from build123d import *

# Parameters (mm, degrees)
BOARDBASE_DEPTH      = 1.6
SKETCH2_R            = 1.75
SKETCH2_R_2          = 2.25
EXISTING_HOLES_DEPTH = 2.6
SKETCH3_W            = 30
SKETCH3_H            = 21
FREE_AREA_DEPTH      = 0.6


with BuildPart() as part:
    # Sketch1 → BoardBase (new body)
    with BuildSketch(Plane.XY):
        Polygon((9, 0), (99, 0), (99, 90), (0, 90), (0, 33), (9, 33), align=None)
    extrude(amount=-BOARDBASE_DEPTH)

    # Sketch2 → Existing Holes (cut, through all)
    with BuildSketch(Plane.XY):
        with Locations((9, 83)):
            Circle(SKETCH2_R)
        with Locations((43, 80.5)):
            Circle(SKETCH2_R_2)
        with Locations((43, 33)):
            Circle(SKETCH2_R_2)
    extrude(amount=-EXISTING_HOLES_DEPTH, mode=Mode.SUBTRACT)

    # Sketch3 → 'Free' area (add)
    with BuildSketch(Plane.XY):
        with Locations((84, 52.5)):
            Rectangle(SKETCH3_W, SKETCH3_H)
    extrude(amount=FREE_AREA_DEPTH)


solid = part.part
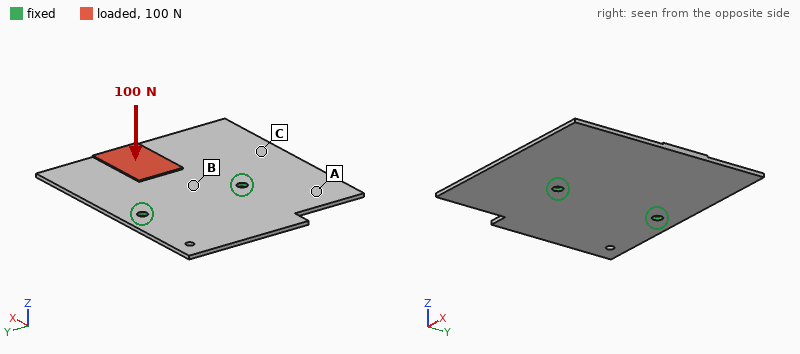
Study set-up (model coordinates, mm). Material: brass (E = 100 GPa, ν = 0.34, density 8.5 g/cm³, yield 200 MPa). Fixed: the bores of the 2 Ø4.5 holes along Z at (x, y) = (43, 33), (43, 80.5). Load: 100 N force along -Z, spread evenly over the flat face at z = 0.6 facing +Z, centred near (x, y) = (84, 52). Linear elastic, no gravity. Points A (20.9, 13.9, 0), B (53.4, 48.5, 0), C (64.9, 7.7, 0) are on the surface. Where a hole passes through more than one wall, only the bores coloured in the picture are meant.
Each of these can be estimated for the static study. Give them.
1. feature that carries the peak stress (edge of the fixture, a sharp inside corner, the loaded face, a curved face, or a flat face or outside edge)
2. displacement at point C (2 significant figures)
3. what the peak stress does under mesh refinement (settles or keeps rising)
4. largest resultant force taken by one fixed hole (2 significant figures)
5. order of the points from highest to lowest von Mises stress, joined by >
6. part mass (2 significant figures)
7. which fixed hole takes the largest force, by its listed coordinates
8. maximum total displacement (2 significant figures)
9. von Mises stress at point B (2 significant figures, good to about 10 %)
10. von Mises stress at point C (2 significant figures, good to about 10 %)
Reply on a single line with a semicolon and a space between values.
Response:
edge of the fixture; 0.25 mm; keeps rising; 57 N; B > C > A; 120 g; (43, 33); 1.4 mm; 75 MPa; 42 MPa
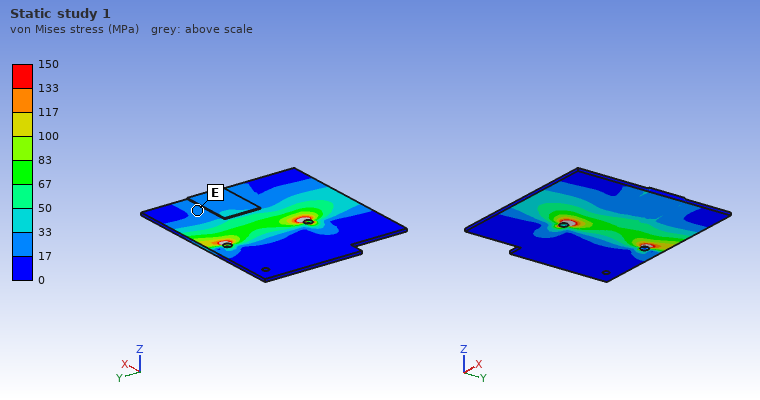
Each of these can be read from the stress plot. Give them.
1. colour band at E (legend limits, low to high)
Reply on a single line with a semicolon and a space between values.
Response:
17 to 33 MPa
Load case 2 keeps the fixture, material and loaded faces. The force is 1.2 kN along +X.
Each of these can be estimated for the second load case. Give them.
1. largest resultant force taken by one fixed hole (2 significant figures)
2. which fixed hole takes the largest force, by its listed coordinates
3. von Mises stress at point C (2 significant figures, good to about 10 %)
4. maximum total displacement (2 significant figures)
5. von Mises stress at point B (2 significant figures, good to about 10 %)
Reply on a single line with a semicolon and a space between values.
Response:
720 N; (43, 33); 27 MPa; 0.82 mm; 52 MPa
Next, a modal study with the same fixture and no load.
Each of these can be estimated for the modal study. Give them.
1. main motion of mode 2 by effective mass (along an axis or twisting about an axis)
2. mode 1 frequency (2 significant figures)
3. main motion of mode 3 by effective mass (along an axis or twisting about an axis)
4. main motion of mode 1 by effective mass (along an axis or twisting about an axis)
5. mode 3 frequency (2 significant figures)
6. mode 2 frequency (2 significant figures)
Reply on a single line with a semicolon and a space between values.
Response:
twisting about X; 250 Hz; along Z; along Z; 510 Hz; 460 Hz
